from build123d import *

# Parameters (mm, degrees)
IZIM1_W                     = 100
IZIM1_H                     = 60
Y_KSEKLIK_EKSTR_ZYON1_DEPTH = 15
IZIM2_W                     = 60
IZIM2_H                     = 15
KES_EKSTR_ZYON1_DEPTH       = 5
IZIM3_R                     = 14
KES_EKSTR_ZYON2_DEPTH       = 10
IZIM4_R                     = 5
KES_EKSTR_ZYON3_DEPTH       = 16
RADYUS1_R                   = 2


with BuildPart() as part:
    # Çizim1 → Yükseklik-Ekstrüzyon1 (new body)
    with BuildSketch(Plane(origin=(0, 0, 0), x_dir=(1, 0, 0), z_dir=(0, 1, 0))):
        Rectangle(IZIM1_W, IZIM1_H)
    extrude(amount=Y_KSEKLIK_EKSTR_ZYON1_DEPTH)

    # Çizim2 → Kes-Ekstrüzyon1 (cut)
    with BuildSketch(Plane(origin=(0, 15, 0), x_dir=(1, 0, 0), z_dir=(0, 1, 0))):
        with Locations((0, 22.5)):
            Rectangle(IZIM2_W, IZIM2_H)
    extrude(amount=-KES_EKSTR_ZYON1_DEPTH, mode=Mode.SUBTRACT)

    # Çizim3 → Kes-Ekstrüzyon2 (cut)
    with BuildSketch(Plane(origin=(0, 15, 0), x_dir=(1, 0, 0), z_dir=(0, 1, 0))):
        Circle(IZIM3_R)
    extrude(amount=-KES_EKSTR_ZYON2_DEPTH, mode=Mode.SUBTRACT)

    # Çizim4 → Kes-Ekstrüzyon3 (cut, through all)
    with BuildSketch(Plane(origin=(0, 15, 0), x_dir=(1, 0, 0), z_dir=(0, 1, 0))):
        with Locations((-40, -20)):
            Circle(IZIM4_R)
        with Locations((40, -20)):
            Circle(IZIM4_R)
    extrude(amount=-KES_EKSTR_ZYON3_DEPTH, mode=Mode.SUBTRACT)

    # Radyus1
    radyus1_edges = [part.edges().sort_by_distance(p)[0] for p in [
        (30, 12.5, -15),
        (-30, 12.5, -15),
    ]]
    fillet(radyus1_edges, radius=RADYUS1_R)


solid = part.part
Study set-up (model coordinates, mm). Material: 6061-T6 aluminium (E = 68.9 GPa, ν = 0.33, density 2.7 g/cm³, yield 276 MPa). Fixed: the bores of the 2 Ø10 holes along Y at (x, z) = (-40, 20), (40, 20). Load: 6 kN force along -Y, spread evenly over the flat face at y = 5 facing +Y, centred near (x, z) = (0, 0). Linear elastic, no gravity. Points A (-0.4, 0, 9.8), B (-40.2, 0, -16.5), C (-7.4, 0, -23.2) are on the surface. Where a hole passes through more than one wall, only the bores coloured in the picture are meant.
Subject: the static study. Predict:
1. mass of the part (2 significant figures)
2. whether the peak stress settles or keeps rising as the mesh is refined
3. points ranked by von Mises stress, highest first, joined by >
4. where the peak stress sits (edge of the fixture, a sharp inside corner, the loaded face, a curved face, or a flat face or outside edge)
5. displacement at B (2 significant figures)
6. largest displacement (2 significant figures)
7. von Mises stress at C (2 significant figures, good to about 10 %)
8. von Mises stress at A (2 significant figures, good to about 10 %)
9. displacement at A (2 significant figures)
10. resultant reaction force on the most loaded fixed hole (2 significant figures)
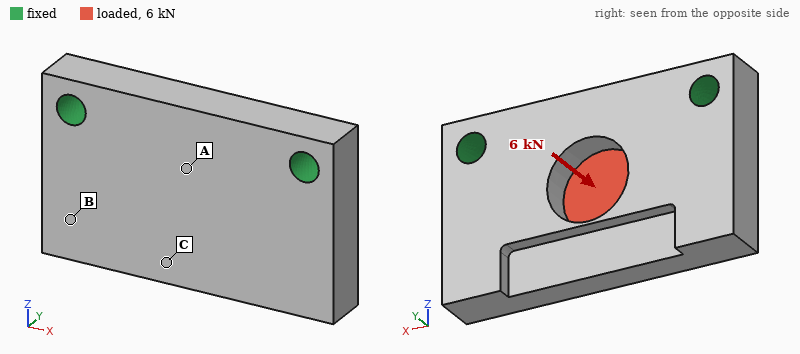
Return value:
210 g
keeps rising
A > C > B
edge of the fixture
36 µm
99 µm
26 MPa
49 MPa
50 µm
3.1 kN
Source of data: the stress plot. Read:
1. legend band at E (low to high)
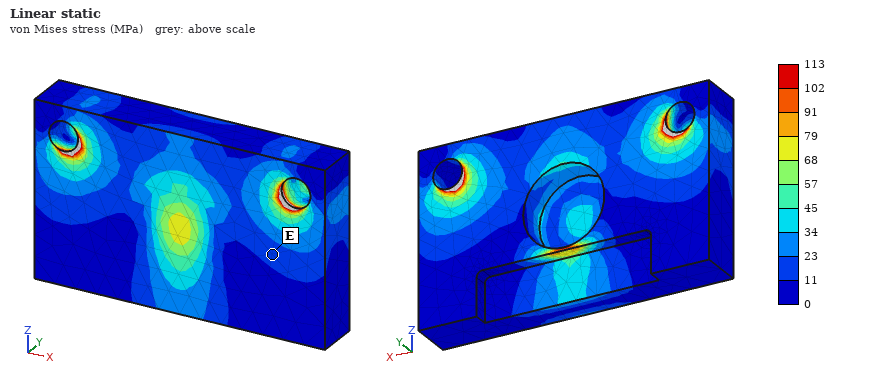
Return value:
11 to 23 MPa
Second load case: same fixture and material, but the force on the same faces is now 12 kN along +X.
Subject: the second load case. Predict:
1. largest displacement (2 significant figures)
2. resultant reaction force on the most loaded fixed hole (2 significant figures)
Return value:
20 µm
6.5 kN
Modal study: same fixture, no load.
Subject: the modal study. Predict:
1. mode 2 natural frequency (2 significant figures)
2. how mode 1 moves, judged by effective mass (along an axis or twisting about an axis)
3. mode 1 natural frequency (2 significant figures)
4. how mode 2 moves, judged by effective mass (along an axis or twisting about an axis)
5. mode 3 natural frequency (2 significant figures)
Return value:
6300 Hz
along Y
4000 Hz
twisting about Z
9200 Hz
